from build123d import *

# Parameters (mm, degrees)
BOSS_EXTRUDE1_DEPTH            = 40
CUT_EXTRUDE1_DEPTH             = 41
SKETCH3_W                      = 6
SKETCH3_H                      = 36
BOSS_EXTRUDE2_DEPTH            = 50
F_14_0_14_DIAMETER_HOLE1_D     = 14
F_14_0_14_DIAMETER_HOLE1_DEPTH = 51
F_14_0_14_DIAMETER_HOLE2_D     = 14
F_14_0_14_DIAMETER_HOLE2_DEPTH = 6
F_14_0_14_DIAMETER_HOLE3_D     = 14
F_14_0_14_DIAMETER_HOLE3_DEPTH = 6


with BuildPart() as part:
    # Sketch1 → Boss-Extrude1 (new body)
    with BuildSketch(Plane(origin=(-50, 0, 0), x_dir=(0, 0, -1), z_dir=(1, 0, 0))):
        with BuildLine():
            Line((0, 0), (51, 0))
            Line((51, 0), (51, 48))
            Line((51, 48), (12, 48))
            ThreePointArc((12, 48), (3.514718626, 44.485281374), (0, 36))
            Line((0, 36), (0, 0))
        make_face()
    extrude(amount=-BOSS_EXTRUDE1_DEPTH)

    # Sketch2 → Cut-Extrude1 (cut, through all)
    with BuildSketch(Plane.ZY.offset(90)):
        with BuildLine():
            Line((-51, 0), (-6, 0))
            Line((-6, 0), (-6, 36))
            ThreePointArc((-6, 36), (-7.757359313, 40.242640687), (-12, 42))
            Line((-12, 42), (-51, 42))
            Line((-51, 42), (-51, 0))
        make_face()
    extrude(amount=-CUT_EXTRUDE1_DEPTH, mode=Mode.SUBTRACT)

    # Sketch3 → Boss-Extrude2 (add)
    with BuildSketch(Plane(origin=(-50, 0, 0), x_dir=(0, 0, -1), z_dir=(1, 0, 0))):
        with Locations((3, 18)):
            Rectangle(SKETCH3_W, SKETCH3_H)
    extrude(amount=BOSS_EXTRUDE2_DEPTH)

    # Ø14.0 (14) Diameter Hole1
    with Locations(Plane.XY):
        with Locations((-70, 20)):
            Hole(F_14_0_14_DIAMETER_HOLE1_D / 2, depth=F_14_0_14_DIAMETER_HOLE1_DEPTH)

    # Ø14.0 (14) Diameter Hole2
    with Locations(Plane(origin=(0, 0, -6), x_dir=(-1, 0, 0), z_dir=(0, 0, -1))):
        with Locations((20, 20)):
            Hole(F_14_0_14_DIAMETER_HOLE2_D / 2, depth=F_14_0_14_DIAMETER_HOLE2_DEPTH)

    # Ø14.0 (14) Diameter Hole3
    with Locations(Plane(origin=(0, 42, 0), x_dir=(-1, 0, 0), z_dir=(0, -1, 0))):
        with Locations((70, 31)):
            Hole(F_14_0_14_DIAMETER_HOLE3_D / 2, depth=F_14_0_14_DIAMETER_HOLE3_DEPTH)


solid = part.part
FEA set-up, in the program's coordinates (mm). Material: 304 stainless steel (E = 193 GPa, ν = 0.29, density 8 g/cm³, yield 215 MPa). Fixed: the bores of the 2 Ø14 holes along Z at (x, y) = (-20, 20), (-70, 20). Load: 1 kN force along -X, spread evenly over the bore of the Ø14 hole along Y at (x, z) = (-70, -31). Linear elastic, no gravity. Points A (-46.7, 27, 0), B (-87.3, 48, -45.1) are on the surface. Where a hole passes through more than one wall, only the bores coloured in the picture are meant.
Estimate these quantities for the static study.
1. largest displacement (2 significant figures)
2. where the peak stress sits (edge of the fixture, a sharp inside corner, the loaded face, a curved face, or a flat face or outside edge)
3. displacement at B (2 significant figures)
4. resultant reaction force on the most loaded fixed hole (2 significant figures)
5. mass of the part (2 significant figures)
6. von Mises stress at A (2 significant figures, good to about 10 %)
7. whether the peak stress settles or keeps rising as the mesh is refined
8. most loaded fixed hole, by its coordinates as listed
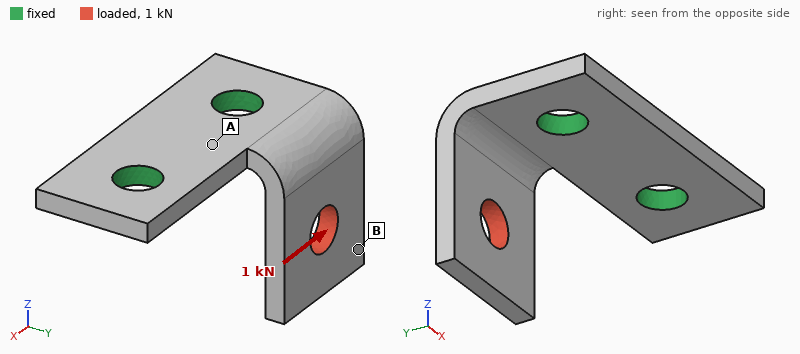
86 µm
edge of the fixture
72 µm
860 N
240 g
35 MPa
keeps rising
(-70, 20)
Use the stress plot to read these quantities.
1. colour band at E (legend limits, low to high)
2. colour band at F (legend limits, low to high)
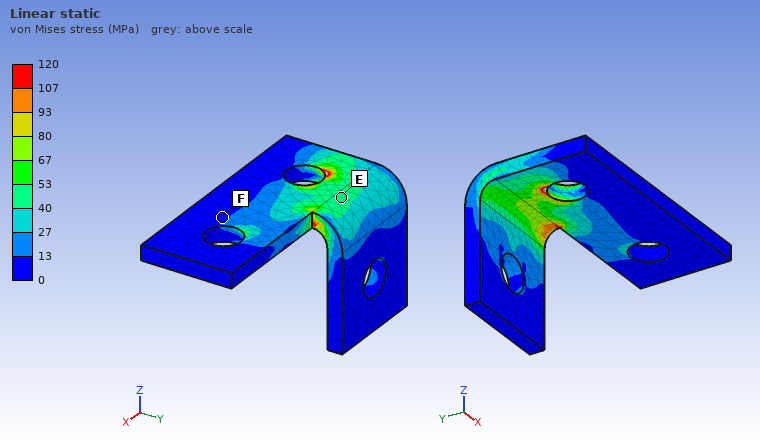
40 to 53 MPa
0 to 13 MPa
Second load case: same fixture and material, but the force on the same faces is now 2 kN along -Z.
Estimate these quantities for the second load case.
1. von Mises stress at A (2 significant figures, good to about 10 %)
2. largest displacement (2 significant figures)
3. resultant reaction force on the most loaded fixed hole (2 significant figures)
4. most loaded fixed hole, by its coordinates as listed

42 MPa
0.15 mm
2.0 kN
(-70, 20)
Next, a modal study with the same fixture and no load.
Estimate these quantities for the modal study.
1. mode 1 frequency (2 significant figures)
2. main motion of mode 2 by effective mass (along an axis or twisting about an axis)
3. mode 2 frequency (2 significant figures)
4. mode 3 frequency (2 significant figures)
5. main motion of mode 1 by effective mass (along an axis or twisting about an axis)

1400 Hz
along X
2400 Hz
5000 Hz
along Y
